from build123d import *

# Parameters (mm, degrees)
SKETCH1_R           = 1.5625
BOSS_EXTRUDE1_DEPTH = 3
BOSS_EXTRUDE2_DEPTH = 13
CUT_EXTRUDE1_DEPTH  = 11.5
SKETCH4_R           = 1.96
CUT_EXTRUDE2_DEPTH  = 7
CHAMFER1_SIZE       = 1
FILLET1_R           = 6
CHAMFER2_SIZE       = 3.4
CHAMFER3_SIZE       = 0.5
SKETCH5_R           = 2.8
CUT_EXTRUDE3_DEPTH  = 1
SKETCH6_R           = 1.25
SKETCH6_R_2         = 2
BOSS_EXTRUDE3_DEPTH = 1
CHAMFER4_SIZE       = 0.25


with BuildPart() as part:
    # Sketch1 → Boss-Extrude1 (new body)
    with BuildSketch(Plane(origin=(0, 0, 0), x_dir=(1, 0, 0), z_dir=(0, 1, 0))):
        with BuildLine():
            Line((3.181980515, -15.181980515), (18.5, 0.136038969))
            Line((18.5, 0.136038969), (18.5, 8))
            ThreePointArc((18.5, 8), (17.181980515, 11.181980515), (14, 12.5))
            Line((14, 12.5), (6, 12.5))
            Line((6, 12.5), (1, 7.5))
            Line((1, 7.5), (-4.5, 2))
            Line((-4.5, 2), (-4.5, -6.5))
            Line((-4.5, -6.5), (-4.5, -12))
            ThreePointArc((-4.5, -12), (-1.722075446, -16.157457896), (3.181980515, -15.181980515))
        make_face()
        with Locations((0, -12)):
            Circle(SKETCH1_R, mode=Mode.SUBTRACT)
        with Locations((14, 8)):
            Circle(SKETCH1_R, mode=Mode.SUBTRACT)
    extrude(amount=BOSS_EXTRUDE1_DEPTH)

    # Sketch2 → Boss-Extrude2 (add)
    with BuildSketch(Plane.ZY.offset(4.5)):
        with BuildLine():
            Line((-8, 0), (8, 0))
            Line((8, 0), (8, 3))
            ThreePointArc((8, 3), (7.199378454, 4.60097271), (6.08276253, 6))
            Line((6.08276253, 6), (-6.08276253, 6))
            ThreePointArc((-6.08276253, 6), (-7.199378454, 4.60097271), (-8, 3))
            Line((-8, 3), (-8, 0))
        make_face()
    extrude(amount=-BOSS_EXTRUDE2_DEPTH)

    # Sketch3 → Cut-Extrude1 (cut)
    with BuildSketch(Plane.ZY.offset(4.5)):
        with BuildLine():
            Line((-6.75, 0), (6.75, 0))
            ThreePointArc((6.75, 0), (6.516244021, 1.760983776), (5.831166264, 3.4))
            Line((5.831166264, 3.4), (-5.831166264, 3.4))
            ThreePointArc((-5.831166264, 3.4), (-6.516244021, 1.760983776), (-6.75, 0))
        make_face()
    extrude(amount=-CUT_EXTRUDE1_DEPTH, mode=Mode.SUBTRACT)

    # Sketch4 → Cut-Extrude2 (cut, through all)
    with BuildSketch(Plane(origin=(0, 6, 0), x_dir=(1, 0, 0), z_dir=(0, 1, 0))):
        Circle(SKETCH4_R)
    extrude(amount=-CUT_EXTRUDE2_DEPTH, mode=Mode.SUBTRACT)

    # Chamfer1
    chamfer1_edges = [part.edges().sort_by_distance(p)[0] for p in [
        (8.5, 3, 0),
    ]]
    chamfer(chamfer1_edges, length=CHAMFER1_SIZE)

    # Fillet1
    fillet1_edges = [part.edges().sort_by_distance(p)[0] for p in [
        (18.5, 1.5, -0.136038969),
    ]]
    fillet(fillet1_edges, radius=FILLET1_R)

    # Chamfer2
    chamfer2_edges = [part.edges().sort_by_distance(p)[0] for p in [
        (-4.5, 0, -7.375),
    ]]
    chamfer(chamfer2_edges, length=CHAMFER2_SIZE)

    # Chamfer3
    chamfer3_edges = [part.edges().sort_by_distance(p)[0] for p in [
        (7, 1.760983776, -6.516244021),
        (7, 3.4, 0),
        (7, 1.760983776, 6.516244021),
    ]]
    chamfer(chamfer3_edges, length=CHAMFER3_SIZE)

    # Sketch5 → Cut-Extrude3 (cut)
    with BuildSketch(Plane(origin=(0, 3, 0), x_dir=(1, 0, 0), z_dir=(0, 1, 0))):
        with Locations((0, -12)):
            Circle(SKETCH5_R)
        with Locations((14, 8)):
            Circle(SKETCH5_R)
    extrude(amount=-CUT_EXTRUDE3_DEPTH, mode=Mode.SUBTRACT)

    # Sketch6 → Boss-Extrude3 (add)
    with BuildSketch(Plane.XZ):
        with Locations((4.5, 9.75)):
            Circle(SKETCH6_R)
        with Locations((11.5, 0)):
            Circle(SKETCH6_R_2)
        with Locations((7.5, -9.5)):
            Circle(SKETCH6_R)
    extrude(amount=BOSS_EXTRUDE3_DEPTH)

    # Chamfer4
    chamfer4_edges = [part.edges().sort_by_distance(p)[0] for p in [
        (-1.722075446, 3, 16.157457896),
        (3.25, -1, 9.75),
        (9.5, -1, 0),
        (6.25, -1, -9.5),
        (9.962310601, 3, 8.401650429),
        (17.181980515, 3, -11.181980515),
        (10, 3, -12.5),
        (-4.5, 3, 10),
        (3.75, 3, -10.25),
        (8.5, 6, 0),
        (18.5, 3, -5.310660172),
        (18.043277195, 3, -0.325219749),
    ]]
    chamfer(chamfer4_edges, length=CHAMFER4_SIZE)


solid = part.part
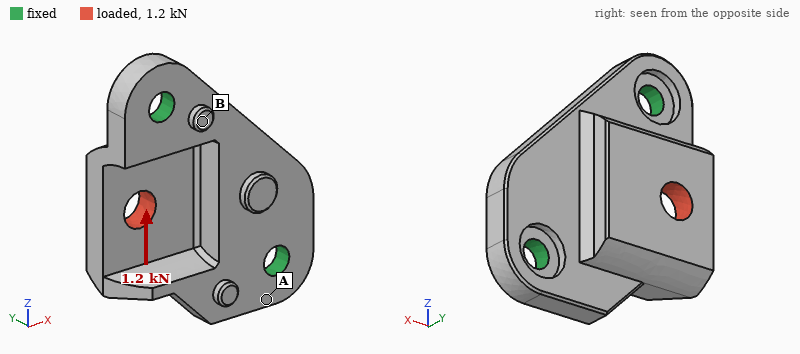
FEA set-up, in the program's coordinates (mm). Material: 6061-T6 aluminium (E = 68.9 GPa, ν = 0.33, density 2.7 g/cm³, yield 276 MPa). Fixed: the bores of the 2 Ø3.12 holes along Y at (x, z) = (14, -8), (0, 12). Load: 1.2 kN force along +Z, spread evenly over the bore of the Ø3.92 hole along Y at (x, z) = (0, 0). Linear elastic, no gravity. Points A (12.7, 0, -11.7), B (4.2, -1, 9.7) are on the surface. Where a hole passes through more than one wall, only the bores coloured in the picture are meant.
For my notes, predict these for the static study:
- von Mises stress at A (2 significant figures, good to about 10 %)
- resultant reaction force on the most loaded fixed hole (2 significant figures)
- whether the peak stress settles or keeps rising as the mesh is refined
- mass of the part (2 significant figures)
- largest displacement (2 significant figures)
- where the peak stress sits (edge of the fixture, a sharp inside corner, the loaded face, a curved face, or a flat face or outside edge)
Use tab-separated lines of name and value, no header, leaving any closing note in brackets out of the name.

von Mises stress at A	71 MPa
resultant reaction force on the most loaded fixed hole	740 N
whether the peak stress settles or keeps rising as the mesh is refined	keeps rising
mass of the part	3.8 g
largest displacement	57 µm
where the peak stress sits	edge of the fixture
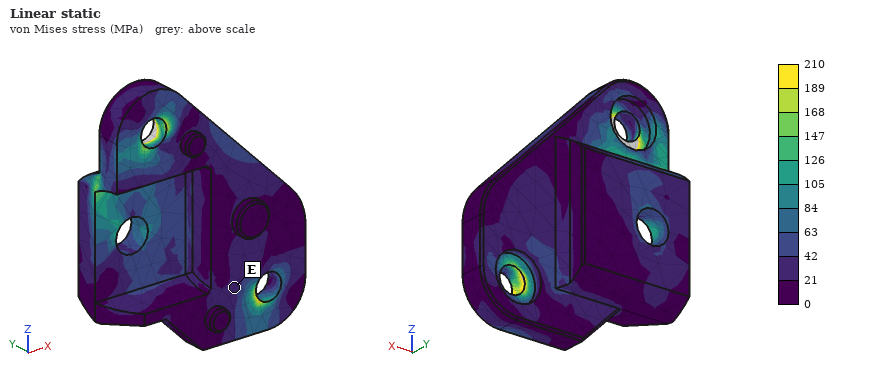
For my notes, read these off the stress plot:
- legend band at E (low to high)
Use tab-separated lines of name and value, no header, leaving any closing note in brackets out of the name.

legend band at E	21 to 42 MPa
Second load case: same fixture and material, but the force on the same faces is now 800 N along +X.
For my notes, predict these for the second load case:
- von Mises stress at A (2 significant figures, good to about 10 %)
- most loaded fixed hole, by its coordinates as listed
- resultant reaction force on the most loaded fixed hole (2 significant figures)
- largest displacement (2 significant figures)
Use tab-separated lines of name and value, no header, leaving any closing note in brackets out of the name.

von Mises stress at A	52 MPa
most loaded fixed hole, by its coordinates as listed	(0, 12)
resultant reaction force on the most loaded fixed hole	450 N
largest displacement	71 µm
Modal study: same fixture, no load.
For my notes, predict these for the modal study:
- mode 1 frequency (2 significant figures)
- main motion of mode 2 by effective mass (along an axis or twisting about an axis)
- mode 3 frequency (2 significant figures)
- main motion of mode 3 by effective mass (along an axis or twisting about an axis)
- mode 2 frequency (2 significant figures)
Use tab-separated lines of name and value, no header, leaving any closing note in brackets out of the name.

mode 1 frequency	11 kHz
main motion of mode 2 by effective mass	along Y
mode 3 frequency	28 kHz
main motion of mode 3 by effective mass	along Z
mode 2 frequency	22 kHz
